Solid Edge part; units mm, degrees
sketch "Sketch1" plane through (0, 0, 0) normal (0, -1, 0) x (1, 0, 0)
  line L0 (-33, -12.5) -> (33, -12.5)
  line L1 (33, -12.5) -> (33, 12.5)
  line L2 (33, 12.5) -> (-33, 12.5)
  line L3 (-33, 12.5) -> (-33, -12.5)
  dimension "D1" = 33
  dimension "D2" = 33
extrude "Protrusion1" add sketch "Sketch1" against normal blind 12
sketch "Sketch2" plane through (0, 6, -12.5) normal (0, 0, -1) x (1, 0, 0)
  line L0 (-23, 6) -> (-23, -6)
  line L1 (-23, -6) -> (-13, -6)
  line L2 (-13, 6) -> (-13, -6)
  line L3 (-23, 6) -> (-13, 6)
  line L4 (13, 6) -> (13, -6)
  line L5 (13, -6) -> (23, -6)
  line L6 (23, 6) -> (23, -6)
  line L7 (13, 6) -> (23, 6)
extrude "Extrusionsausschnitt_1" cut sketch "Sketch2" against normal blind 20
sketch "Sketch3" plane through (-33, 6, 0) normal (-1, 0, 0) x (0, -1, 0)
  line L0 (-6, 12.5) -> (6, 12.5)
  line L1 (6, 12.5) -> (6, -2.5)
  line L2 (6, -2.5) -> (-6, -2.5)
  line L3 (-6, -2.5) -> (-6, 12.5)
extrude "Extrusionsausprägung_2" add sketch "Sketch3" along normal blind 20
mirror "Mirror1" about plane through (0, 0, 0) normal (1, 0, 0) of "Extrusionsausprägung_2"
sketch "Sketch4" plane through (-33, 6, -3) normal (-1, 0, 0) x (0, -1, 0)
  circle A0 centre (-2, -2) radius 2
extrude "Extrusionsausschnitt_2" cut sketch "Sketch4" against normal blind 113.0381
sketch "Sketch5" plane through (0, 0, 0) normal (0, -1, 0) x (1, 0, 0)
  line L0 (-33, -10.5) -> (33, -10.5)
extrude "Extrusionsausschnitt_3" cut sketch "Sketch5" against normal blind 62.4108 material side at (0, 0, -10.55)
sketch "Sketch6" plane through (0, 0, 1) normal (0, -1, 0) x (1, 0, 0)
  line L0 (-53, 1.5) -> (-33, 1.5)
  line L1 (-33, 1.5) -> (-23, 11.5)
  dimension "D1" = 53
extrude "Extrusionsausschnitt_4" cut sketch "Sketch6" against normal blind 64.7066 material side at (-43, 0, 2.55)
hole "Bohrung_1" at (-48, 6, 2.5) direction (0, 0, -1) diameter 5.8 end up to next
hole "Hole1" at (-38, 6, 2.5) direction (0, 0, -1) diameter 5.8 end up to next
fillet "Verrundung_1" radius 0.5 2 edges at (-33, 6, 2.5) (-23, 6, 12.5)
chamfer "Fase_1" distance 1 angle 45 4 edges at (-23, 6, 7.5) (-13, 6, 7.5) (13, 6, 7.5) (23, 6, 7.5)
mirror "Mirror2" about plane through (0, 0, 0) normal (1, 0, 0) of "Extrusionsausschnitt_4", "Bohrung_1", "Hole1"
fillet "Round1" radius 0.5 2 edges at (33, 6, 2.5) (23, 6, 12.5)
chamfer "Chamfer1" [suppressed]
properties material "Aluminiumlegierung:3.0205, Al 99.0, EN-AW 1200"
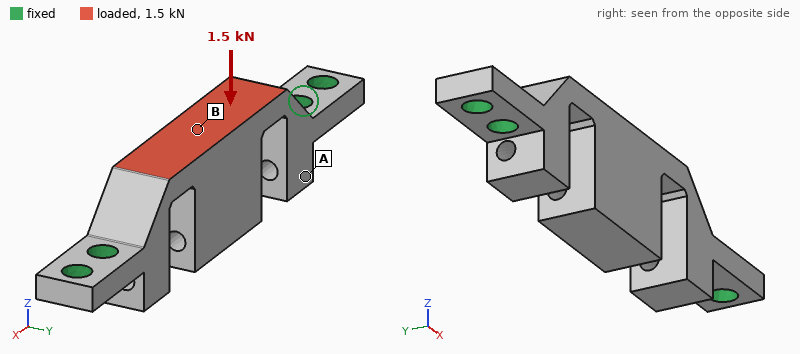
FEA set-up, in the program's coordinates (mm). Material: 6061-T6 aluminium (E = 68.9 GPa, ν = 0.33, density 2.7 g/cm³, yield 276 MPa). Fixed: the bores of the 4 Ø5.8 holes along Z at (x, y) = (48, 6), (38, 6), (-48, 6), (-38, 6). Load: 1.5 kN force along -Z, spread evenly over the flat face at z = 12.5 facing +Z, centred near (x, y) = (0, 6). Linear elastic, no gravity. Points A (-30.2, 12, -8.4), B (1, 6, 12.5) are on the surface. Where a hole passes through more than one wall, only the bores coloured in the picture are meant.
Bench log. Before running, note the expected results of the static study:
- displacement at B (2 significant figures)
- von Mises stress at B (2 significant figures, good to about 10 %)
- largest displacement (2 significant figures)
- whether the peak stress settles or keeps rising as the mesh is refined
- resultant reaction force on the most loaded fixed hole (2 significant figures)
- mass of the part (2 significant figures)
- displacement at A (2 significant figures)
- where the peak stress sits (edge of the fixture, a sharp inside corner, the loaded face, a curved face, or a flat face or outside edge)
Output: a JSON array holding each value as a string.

["44 µm", "26 MPa", "44 µm", "keeps rising", "1.2 kN", "38 g", "10 µm", "edge of the fixture"]
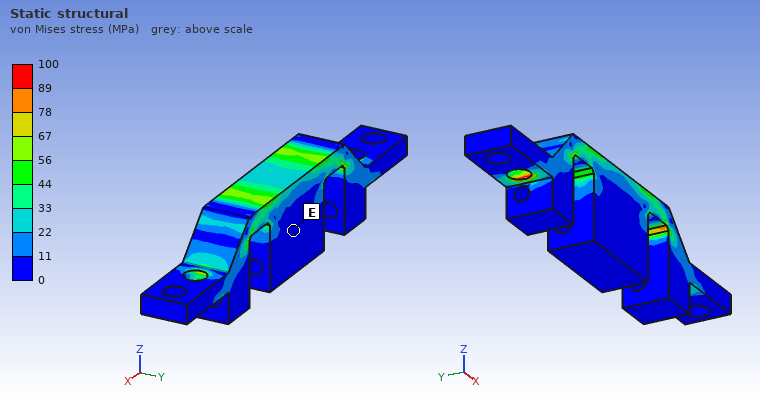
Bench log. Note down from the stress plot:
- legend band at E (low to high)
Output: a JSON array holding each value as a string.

["0 to 11 MPa"]
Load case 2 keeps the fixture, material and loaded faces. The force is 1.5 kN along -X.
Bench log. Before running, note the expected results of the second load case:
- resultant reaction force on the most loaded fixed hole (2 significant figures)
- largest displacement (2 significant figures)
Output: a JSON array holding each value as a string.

["730 N", "51 µm"]
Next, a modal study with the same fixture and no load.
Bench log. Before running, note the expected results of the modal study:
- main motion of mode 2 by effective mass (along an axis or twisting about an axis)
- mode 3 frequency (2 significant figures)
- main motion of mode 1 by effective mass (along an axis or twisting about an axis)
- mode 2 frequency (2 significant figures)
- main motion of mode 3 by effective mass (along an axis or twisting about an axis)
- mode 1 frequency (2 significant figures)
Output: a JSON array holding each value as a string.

["along X", "6000 Hz", "along Y", "4500 Hz", "along Z", "3400 Hz"]
